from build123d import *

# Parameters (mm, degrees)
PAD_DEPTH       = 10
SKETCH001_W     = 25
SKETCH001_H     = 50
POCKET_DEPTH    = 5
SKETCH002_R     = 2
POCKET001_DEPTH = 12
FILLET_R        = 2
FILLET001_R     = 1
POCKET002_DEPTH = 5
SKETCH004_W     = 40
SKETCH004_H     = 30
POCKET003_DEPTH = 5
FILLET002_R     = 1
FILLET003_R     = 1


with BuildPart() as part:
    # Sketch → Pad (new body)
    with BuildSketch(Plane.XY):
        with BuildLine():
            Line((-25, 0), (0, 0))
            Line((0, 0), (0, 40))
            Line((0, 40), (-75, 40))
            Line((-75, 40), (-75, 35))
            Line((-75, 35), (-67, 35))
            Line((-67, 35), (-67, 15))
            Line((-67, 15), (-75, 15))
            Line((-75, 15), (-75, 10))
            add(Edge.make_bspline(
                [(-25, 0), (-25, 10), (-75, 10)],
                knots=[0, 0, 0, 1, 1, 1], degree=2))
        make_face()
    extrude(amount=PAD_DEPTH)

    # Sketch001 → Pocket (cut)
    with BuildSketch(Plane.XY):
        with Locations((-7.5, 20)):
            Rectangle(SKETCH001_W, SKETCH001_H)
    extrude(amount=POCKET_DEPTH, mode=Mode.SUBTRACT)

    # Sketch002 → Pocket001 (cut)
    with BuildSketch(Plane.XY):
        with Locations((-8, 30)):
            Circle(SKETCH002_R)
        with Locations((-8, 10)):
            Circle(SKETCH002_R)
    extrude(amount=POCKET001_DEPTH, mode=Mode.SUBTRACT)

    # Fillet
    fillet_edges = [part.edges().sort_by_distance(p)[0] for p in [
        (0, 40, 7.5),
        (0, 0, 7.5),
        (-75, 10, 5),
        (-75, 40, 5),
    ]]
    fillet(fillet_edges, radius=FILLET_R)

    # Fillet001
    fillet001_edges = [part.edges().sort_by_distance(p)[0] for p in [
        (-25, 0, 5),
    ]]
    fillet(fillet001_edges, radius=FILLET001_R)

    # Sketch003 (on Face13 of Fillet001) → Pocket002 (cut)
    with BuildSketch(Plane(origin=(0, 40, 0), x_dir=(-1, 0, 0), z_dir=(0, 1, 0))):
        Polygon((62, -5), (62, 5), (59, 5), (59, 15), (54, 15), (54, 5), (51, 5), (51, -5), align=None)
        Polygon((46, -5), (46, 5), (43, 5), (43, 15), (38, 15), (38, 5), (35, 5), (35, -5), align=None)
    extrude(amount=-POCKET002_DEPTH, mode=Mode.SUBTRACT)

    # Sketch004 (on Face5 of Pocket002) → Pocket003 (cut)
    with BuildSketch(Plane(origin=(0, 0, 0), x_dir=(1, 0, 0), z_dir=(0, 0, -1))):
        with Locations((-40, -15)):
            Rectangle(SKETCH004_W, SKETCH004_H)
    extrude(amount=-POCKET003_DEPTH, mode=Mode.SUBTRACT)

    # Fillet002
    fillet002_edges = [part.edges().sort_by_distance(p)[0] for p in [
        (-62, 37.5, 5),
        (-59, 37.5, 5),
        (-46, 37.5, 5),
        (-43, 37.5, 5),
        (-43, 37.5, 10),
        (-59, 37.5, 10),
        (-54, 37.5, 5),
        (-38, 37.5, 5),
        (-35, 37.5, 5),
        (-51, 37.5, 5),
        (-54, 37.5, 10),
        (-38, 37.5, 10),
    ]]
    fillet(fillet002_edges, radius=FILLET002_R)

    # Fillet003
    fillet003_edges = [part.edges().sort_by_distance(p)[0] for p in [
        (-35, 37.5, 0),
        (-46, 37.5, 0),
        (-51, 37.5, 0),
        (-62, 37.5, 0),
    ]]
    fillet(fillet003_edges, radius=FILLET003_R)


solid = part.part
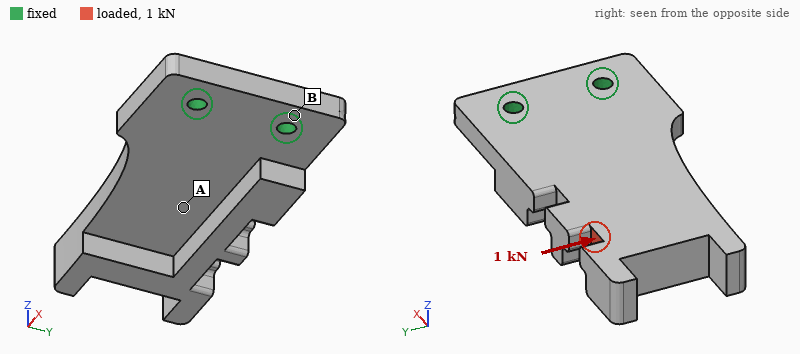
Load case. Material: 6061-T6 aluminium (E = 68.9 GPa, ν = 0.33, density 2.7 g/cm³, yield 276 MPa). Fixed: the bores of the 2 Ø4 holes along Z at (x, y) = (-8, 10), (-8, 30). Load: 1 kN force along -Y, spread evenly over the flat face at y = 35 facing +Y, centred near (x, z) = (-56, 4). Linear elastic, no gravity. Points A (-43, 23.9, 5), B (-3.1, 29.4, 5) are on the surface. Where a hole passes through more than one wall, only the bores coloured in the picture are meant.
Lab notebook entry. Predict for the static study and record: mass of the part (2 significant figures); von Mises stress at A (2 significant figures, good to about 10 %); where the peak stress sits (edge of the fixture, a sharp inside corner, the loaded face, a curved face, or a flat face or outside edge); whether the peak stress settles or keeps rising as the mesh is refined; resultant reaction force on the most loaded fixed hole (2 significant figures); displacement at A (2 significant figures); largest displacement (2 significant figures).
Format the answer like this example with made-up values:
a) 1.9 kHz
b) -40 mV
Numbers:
a) 39 g
b) 34 MPa
c) edge of the fixture
d) keeps rising
e) 2.2 kN
f) 0.036 mm
g) 0.13 mm
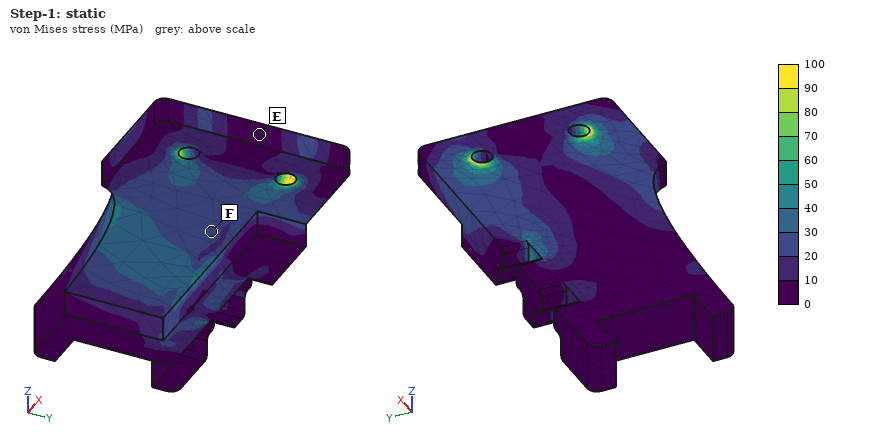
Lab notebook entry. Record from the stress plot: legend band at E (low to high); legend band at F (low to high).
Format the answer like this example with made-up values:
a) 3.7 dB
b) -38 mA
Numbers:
a) 0 to 10 MPa
b) 20 to 30 MPa
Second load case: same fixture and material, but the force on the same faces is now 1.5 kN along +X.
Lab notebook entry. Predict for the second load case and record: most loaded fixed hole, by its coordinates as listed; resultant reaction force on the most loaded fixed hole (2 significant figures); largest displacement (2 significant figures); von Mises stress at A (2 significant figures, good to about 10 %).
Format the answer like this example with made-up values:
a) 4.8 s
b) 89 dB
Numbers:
a) (-8, 30)
b) 1.8 kN
c) 0.25 mm
d) 13 MPa
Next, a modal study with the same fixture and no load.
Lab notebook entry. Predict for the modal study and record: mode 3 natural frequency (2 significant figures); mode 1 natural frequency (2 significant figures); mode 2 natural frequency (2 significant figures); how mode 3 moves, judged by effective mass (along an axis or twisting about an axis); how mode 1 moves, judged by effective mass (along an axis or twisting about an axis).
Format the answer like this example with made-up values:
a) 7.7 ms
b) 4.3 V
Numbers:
a) 5000 Hz
b) 1000 Hz
c) 3900 Hz
d) along Y
e) along Z
